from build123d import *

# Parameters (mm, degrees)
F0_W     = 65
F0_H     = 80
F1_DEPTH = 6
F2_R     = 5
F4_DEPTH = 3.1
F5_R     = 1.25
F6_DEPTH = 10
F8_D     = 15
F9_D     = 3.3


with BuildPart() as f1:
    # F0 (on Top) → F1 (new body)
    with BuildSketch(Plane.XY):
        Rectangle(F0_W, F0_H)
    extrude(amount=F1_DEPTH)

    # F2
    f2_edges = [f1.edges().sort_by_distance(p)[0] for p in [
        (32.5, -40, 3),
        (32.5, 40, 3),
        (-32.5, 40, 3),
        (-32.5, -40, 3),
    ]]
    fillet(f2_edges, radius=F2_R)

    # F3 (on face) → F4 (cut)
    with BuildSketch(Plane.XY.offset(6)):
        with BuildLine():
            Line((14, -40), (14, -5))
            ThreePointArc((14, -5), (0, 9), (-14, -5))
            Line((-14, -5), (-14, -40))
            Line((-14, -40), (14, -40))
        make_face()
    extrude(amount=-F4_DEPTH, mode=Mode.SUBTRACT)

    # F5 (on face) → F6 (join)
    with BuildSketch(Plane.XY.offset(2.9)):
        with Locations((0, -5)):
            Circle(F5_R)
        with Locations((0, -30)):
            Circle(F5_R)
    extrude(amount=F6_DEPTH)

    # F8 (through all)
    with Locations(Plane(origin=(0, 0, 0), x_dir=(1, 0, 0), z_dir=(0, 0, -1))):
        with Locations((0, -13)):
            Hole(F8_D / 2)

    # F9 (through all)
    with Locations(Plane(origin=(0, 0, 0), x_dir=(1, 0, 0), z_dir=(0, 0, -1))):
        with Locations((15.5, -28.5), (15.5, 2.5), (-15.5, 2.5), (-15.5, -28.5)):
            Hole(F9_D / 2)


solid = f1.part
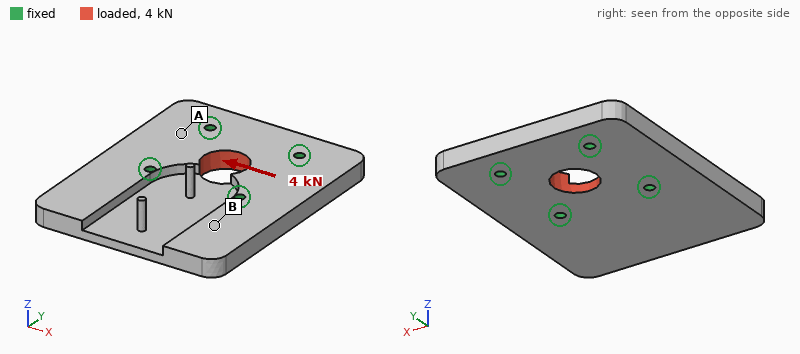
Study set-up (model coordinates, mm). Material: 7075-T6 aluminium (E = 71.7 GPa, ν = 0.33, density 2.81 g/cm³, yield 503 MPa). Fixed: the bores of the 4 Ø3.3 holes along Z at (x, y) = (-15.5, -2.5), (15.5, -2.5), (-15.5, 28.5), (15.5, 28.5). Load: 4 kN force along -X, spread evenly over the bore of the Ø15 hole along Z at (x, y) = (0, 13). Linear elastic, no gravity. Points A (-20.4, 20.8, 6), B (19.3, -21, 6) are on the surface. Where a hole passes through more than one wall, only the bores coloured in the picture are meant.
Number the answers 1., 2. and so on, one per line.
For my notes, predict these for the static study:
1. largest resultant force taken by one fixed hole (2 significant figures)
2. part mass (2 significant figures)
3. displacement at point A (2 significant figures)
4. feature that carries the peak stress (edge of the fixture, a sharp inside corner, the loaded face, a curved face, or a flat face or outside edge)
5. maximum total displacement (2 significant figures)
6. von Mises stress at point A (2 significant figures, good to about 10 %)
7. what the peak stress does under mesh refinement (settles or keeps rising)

1. 1.2 kN
2. 73 g
3. 2.2 µm
4. edge of the fixture
5. 4.9 µm
6. 8.4 MPa
7. keeps rising
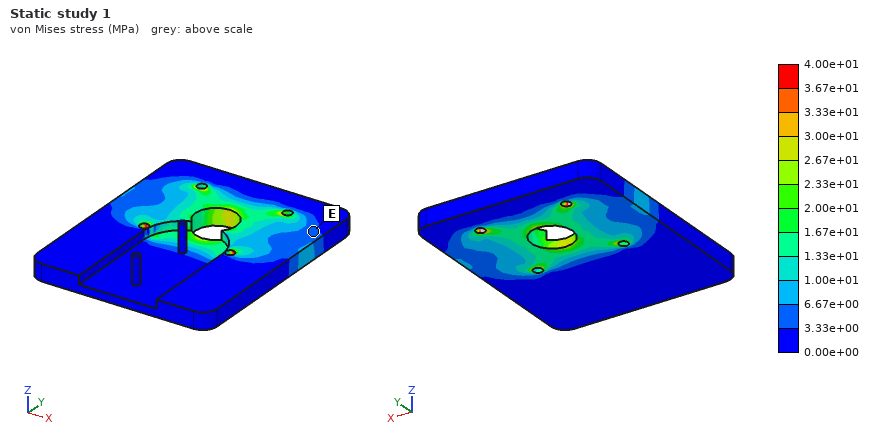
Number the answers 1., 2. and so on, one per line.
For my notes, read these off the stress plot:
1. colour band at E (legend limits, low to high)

1. 3.33e+00 to 6.67e+00 MPa
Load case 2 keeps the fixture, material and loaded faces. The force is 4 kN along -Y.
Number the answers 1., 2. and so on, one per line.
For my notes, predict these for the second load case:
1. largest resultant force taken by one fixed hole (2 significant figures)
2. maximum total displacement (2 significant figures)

1. 1.2 kN
2. 6.4 µm
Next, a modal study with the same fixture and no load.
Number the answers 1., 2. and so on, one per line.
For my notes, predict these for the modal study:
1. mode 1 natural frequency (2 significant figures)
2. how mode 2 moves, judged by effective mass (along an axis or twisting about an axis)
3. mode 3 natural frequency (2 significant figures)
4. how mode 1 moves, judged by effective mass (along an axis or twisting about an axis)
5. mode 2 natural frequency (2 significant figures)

1. 2900 Hz
2. twisting about Y
3. 7100 Hz
4. along Z
5. 3700 Hz
